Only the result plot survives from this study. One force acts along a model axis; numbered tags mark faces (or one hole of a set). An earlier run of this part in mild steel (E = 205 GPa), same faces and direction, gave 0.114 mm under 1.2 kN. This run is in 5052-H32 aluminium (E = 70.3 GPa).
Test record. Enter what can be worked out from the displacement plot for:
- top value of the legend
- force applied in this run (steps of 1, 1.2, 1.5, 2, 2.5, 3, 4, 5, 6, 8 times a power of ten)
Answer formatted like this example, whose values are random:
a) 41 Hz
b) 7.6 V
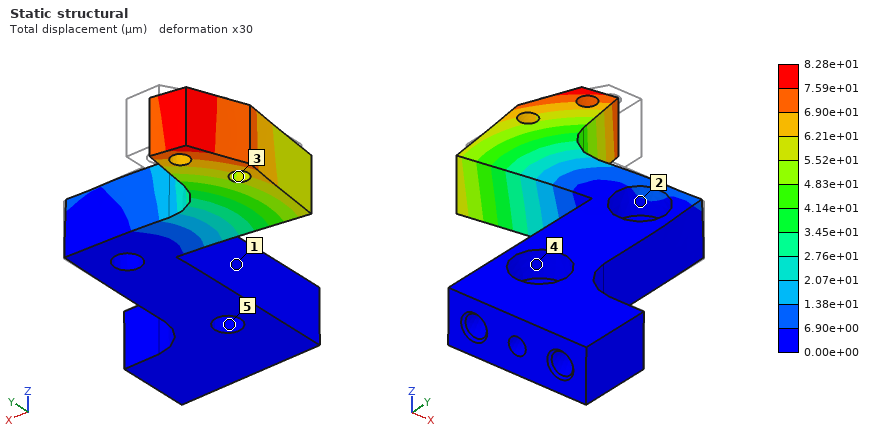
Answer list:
a) 8.28e+01 µm
b) 300 N
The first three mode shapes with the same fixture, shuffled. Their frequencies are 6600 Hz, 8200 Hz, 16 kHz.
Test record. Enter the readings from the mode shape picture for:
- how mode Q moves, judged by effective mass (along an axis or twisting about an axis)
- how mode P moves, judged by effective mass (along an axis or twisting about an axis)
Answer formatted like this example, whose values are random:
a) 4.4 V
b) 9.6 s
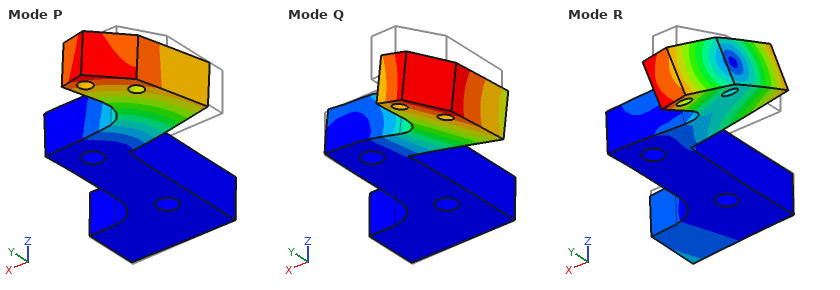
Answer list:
a) along Z
b) along Y
